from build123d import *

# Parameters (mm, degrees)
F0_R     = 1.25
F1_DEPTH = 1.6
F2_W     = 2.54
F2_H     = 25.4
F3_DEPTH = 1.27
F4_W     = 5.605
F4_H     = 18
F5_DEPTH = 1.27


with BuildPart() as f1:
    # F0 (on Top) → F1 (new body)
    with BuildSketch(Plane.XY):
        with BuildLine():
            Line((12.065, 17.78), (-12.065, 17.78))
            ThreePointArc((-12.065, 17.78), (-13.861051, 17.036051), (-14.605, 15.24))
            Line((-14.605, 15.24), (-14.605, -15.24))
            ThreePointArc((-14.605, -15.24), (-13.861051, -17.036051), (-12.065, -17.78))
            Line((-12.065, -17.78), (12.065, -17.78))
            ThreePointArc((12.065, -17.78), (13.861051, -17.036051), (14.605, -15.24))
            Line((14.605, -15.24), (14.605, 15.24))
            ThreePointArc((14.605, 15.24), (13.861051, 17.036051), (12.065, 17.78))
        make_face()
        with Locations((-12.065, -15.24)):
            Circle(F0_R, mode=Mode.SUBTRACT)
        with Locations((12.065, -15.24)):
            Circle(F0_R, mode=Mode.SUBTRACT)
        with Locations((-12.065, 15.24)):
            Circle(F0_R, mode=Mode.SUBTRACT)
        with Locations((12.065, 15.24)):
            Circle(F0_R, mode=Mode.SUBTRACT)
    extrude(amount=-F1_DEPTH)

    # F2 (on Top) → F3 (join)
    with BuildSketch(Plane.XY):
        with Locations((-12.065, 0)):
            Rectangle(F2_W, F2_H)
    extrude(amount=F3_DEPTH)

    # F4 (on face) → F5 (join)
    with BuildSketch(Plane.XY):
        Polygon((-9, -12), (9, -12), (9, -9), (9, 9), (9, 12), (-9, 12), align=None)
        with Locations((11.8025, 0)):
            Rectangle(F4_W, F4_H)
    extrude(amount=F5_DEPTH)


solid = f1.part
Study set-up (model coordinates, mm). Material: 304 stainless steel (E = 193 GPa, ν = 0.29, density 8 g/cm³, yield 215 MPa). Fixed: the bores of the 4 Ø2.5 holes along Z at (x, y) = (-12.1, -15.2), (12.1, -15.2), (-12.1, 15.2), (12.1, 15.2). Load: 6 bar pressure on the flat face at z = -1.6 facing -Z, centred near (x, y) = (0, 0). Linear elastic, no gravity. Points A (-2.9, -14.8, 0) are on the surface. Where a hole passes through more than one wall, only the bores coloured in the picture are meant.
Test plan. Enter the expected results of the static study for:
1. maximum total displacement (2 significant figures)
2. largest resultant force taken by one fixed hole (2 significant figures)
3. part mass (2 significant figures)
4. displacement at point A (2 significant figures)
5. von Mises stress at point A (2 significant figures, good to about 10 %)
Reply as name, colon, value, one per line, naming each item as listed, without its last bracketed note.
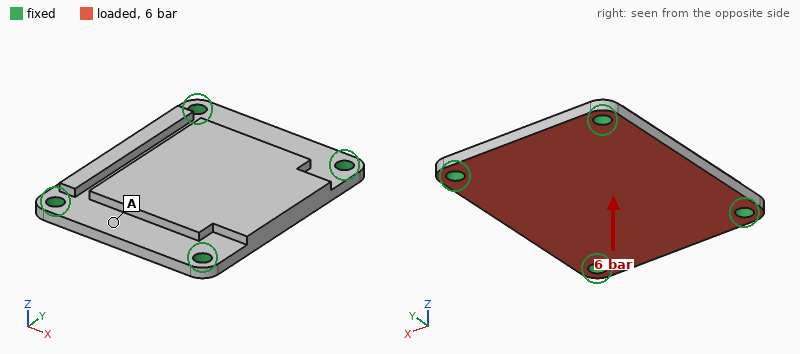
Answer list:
maximum total displacement: 12 µm
largest resultant force taken by one fixed hole: 200 N
part mass: 19 g
displacement at point A: 6.0 µm
von Mises stress at point A: 20 MPa
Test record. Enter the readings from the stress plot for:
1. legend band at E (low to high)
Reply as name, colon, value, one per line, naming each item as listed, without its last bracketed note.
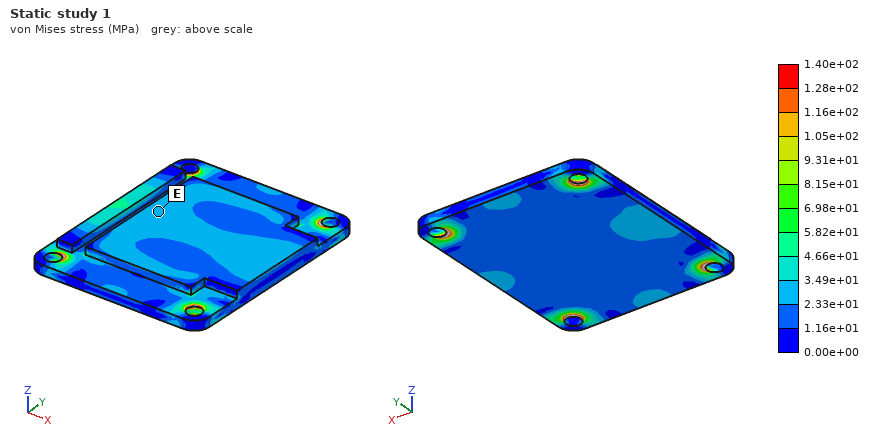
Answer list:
legend band at E: 2.33e+01 to 3.49e+01 MPa
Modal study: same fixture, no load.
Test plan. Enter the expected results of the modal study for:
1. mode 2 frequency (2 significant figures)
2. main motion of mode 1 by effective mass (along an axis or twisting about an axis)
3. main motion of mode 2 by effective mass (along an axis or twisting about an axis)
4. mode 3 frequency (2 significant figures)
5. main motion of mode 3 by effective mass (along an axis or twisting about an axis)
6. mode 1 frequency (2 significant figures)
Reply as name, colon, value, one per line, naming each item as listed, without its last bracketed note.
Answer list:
mode 2 frequency: 14 kHz
main motion of mode 1 by effective mass: along Z
main motion of mode 2 by effective mass: twisting about Y
mode 3 frequency: 17 kHz
main motion of mode 3 by effective mass: twisting about X
mode 1 frequency: 9000 Hz
